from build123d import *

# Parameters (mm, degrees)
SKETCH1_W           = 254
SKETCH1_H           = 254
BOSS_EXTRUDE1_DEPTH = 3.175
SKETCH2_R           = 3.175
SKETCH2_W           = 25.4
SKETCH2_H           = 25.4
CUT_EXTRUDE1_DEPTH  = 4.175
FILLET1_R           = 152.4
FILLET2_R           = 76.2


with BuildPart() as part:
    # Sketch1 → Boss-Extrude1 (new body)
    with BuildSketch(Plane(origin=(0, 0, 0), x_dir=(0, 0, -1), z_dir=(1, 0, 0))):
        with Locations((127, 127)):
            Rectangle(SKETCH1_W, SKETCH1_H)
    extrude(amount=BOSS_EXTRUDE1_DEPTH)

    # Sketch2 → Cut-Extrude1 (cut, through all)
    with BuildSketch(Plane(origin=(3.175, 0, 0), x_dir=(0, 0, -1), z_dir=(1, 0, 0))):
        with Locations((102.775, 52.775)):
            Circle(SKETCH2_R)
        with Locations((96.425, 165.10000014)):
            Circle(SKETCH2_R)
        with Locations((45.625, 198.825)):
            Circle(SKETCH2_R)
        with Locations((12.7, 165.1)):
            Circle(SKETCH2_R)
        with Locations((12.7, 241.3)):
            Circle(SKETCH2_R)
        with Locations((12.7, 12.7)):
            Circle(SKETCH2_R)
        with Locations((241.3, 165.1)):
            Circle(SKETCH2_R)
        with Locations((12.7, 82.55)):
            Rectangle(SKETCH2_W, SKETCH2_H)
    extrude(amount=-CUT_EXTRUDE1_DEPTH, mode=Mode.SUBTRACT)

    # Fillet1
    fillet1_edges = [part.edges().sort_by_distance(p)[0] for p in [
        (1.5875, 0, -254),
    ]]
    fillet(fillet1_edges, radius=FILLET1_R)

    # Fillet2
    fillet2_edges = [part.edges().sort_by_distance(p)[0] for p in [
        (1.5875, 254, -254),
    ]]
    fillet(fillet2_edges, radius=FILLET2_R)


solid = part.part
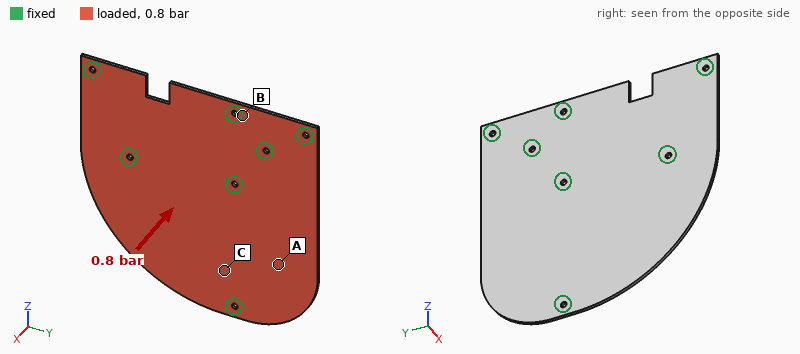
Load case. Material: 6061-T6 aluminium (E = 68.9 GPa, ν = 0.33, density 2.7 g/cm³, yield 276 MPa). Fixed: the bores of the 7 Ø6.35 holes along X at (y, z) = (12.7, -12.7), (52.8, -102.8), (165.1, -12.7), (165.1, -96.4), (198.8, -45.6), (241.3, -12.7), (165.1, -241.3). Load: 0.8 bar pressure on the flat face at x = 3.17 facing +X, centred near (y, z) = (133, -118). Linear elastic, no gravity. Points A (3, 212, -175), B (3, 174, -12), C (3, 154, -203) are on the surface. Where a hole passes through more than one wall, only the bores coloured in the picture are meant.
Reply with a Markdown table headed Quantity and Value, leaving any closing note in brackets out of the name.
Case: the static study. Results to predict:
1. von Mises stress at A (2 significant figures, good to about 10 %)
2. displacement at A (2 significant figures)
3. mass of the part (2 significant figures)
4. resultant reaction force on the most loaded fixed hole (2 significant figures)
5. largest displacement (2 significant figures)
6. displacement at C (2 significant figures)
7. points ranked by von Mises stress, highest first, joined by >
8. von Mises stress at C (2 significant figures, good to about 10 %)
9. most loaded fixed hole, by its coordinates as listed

| Quantity | Value |
|---|---|
| von Mises stress at A | 59 MPa |
| displacement at A | 1.8 mm |
| mass of the part | 490 g |
| resultant reaction force on the most loaded fixed hole | 1.3 kN |
| largest displacement | 3.2 mm |
| displacement at C | 0.64 mm |
| points ranked by von Mises stress, highest first, joined by > | C > A > B |
| von Mises stress at C | 97 MPa |
| most loaded fixed hole, by its coordinates as listed | (52.8, -102.8) |
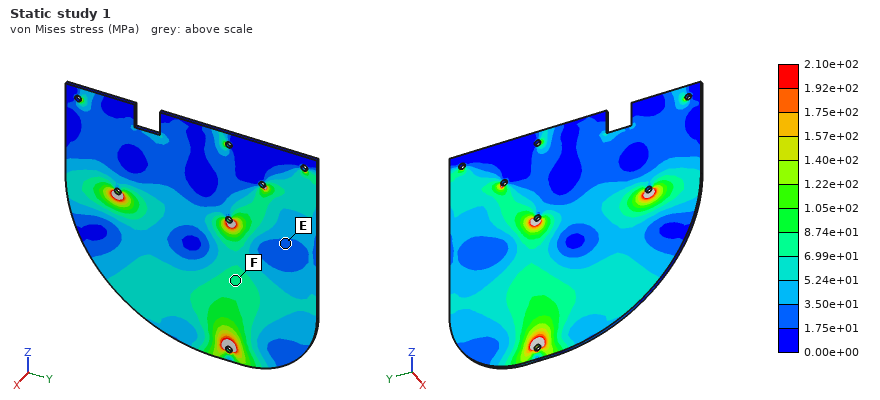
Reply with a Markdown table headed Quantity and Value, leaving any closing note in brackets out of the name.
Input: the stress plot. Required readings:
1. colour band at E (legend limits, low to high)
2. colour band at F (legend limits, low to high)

| Quantity | Value |
|---|---|
| colour band at E | 1.75e+01 to 3.50e+01 MPa |
| colour band at F | 6.99e+01 to 8.74e+01 MPa |
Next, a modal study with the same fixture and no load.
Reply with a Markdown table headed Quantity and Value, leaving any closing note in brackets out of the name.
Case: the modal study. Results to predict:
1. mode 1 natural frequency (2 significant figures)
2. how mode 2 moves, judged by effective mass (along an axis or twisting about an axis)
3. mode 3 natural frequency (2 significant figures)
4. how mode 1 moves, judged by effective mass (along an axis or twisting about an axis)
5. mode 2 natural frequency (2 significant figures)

| Quantity | Value |
|---|---|
| mode 1 natural frequency | 330 Hz |
| how mode 2 moves, judged by effective mass | along X |
| mode 3 natural frequency | 730 Hz |
| how mode 1 moves, judged by effective mass | twisting about Z |
| mode 2 natural frequency | 370 Hz |
